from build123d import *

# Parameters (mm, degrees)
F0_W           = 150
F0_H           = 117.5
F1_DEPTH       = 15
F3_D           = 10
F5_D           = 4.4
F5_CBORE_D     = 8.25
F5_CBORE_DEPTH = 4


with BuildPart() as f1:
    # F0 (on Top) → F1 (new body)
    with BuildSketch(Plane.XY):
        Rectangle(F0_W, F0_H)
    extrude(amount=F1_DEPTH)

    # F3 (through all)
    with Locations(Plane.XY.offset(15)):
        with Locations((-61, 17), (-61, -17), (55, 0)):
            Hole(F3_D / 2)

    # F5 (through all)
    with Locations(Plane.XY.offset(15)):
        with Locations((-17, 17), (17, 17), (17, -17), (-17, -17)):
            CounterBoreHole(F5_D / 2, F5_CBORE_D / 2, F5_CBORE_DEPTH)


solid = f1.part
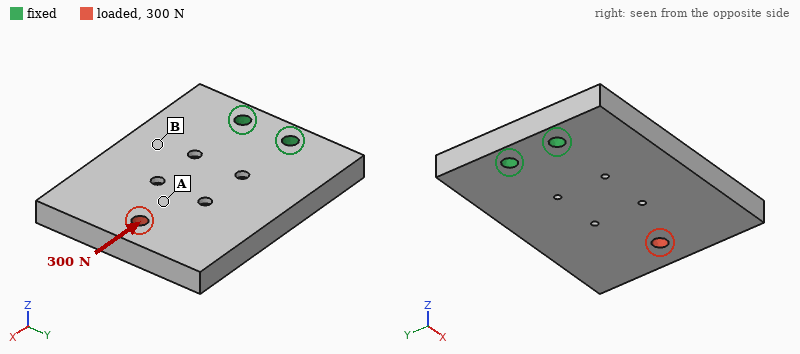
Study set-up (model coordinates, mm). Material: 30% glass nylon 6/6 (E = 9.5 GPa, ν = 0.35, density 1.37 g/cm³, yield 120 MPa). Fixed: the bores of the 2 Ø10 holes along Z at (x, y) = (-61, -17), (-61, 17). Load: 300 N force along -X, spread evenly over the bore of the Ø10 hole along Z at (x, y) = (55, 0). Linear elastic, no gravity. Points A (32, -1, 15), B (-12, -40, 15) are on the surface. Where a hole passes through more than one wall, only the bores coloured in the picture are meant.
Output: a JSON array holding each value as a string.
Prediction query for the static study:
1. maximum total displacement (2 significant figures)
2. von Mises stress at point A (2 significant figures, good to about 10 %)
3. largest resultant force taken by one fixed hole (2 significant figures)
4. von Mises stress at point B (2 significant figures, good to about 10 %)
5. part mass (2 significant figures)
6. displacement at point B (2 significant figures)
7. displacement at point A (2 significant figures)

["4.7 µm", "0.45 MPa", "150 N", "0.15 MPa", "360 g", "1.6 µm", "3.0 µm"]
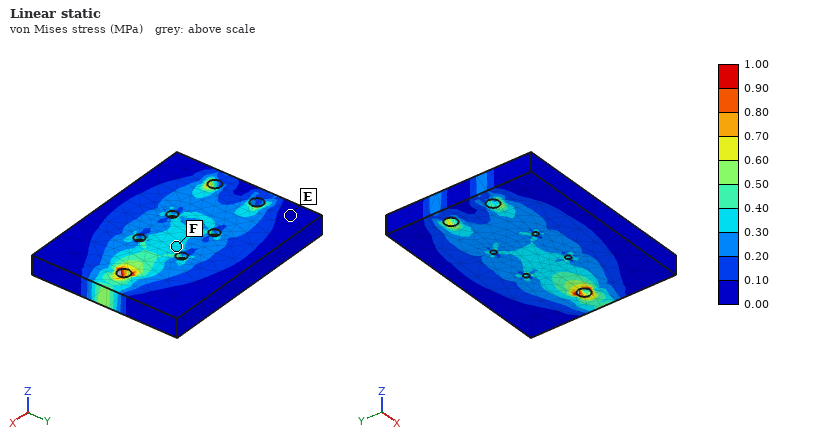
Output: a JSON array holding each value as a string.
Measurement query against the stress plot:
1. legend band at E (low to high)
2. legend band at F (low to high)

["0.00 to 0.10 MPa", "0.30 to 0.40 MPa"]
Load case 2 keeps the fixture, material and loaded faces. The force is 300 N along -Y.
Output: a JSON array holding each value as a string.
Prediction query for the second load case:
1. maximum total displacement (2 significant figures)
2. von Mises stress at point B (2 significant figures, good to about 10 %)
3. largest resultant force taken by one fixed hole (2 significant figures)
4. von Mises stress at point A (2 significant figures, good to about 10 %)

["53 µm", "0.44 MPa", "810 N", "0.43 MPa"]
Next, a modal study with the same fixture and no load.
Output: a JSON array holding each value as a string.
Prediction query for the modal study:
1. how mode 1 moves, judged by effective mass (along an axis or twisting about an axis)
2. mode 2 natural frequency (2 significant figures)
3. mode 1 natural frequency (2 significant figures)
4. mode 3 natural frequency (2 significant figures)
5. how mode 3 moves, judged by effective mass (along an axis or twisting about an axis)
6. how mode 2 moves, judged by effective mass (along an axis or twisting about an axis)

["along Z", "770 Hz", "330 Hz", "1000 Hz", "along Y", "twisting about X"]
